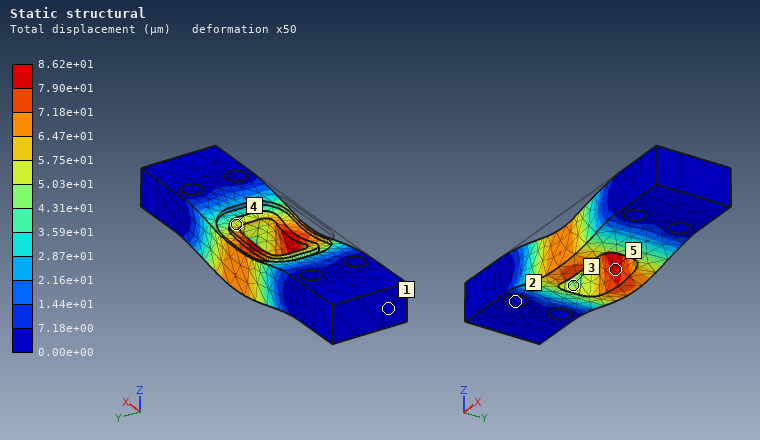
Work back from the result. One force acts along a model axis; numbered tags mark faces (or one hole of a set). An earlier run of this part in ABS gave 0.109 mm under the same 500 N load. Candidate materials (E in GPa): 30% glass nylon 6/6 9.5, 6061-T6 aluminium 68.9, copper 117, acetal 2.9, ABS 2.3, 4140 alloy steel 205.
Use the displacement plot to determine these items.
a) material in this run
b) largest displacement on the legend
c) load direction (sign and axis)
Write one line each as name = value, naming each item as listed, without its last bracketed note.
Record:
material in this run = acetal
largest displacement on the legend = 8.62e+01 µm
load direction = -Z
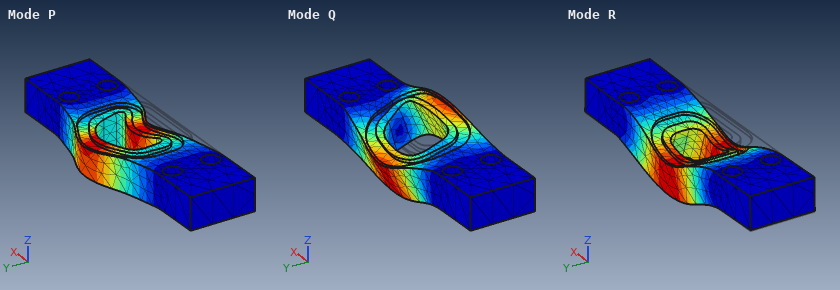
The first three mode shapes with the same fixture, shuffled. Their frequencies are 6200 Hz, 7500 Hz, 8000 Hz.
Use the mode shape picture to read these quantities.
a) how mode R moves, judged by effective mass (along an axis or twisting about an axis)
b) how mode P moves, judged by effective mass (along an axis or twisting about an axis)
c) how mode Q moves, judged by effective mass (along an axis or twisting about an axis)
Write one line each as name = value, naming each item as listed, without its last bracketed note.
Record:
how mode R moves, judged by effective mass = along Z
how mode P moves, judged by effective mass = along Y
how mode Q moves, judged by effective mass = twisting about X
